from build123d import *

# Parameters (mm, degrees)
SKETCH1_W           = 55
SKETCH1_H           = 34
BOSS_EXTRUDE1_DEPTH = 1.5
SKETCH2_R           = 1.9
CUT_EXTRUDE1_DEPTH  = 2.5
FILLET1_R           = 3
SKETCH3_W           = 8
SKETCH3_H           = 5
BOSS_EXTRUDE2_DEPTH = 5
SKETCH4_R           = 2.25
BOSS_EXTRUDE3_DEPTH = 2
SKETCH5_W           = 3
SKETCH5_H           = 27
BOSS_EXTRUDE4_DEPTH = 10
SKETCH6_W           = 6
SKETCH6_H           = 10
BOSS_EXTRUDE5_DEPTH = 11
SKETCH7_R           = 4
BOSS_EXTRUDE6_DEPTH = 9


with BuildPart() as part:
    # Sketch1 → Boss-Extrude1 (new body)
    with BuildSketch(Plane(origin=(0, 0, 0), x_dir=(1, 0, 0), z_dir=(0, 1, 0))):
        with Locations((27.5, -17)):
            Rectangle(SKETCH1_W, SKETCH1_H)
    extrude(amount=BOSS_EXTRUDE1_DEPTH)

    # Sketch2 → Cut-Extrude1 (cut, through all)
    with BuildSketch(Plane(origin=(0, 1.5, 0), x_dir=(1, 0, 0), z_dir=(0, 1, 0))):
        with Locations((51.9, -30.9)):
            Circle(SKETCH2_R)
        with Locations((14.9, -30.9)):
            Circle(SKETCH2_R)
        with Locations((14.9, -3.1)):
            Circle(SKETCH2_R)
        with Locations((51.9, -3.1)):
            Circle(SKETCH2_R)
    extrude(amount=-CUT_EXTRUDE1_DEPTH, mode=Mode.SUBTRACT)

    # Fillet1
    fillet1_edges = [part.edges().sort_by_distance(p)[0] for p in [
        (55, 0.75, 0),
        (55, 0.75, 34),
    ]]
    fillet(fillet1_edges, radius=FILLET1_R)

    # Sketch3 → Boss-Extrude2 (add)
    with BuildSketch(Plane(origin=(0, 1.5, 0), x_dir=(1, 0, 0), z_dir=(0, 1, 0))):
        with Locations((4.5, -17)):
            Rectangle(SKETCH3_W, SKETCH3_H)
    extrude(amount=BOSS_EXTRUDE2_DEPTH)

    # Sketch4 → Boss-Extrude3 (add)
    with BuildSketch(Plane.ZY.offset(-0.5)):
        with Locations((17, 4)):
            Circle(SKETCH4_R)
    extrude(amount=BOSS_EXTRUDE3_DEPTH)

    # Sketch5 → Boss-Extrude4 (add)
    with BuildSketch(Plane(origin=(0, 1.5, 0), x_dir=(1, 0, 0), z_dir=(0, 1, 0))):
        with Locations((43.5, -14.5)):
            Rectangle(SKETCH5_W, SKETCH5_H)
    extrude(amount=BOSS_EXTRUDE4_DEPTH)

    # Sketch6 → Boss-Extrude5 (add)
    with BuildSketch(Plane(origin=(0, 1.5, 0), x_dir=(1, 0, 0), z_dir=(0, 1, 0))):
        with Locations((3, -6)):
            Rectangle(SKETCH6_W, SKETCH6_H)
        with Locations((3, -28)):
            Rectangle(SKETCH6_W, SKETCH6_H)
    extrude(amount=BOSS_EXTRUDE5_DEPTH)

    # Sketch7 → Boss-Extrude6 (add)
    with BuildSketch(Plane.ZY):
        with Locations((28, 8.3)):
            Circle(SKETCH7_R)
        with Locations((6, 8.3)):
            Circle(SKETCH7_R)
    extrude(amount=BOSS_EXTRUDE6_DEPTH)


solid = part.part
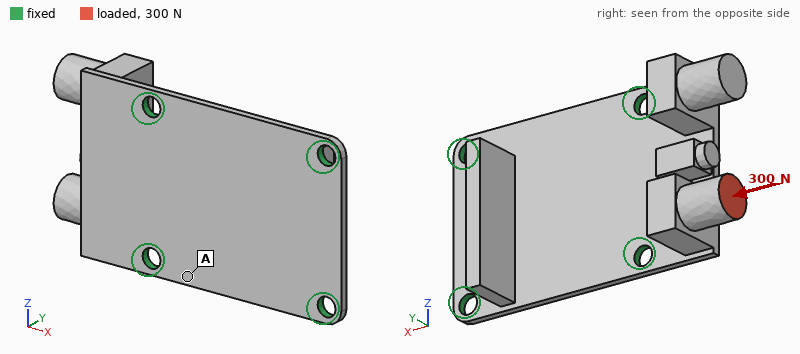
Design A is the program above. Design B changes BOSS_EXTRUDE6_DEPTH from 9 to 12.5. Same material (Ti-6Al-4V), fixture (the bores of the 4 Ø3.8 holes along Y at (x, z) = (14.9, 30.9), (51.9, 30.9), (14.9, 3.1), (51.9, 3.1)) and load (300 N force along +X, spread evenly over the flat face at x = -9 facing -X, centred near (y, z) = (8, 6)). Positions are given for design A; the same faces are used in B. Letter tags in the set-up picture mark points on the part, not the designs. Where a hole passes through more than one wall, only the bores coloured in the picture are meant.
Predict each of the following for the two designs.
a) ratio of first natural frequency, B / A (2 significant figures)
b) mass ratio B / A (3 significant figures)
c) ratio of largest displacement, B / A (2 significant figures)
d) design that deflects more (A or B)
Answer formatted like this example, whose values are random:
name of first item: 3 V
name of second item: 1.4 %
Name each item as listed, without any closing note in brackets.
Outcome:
ratio of first natural frequency, B / A: 0.84
mass ratio B / A: 1.06
ratio of largest displacement, B / A: 1.1
design that deflects more: B
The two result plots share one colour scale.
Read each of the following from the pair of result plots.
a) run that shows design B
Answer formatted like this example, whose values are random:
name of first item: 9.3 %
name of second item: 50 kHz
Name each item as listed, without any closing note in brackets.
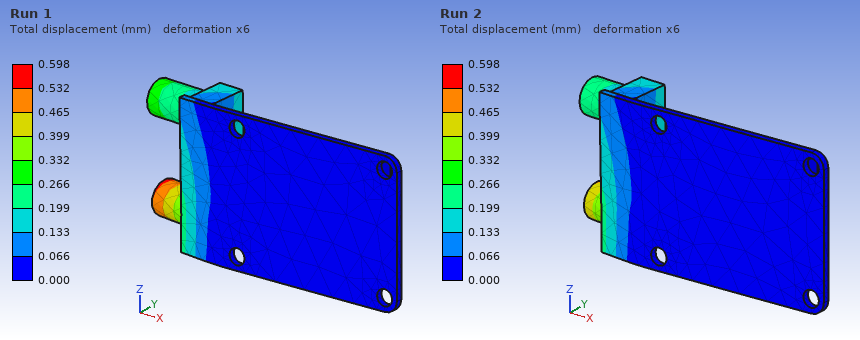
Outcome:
run that shows design B: Run 1
